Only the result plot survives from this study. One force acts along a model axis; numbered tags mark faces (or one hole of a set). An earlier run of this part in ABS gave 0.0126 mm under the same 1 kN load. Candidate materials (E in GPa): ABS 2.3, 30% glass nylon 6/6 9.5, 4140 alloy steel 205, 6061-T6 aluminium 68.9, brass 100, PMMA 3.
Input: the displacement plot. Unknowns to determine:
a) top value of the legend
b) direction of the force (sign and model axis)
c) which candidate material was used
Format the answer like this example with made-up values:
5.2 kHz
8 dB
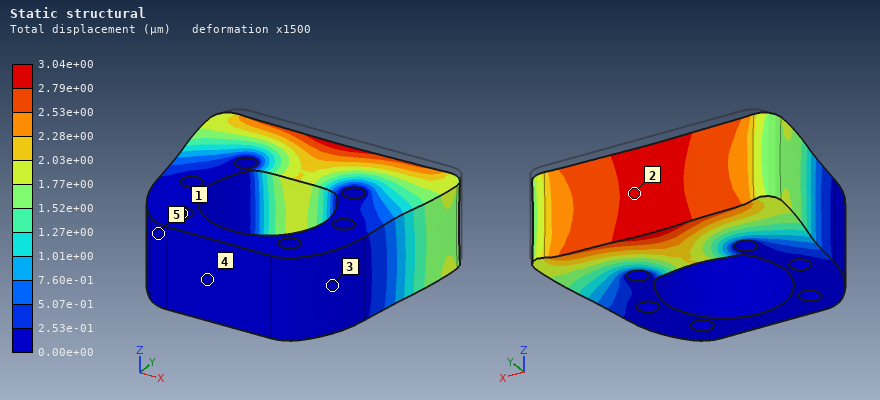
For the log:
3.04e+00 µm
-Y
30% glass nylon 6/6
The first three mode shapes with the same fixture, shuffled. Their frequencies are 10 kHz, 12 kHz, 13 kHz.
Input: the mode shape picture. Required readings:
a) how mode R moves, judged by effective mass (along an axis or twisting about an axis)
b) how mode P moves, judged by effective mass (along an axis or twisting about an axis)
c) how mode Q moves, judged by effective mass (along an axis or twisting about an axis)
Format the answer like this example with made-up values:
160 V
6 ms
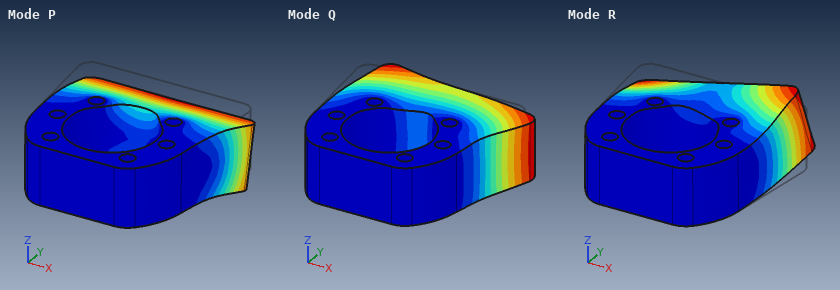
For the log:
twisting about Y
along Z
along X
